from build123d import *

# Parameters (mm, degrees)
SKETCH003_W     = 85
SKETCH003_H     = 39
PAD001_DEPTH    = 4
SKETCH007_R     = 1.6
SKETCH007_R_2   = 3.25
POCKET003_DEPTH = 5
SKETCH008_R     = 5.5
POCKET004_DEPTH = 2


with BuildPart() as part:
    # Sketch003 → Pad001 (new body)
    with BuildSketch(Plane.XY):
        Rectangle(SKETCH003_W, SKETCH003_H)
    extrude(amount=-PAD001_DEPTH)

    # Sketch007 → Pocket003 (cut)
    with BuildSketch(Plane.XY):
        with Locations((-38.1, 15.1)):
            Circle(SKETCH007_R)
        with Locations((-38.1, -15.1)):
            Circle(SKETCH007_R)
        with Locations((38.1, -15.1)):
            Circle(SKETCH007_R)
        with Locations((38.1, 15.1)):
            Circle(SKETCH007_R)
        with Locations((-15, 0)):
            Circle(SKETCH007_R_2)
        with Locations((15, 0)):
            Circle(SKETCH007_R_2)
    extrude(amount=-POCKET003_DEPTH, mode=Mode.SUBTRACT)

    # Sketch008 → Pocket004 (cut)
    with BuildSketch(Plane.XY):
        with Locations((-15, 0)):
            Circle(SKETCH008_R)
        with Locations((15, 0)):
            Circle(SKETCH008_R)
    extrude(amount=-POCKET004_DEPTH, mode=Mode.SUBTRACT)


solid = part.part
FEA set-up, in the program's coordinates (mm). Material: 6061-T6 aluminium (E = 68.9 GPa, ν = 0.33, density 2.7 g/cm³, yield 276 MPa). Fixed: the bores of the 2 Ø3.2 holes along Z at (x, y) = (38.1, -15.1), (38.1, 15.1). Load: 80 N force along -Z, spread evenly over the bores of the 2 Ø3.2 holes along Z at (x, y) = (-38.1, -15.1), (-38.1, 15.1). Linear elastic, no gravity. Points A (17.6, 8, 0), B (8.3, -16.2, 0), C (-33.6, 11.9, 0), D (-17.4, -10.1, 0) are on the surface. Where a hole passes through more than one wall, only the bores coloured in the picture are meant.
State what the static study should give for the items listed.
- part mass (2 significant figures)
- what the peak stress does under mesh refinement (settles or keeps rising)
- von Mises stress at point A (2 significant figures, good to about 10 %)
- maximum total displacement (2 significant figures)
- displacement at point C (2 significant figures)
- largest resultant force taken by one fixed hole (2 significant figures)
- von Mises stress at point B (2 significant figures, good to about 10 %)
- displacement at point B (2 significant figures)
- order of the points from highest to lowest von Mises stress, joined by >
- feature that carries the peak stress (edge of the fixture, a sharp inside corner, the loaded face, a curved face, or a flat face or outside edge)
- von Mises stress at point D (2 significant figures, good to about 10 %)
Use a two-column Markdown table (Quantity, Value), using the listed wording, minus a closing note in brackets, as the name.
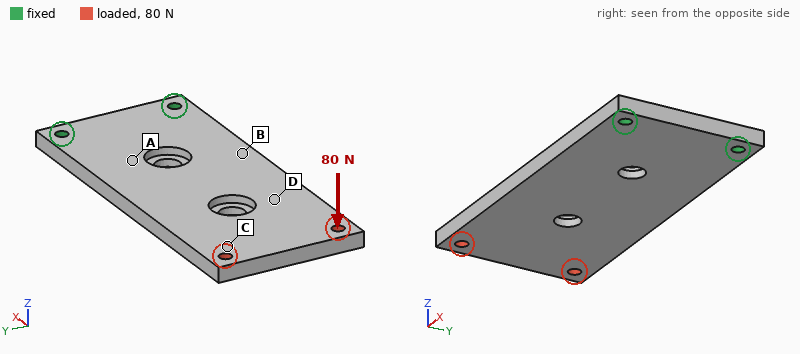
| Quantity | Value |
|---|---|
| part mass | 34 g |
| what the peak stress does under mesh refinement | keeps rising |
| von Mises stress at point A | 57 MPa |
| maximum total displacement | 1.0 mm |
| displacement at point C | 0.88 mm |
| largest resultant force taken by one fixed hole | 44 N |
| von Mises stress at point B | 42 MPa |
| displacement at point B | 0.20 mm |
| order of the points from highest to lowest von Mises stress, joined by > | A > B > D > C |
| feature that carries the peak stress | edge of the fixture |
| von Mises stress at point D | 21 MPa |
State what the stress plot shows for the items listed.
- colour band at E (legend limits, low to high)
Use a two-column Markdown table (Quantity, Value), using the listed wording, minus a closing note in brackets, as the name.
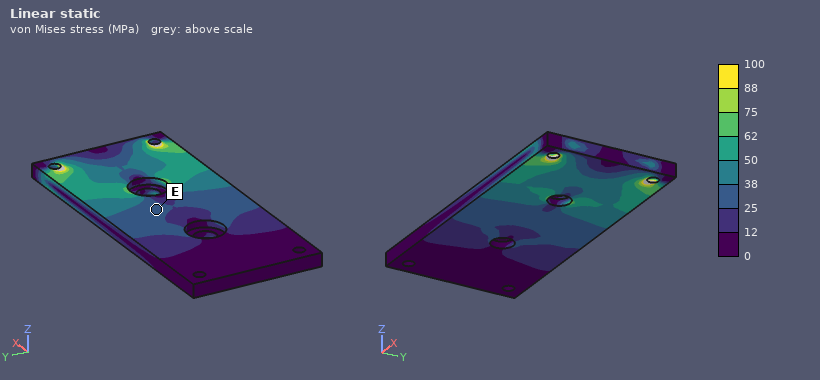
| Quantity | Value |
|---|---|
| colour band at E | 25 to 38 MPa |
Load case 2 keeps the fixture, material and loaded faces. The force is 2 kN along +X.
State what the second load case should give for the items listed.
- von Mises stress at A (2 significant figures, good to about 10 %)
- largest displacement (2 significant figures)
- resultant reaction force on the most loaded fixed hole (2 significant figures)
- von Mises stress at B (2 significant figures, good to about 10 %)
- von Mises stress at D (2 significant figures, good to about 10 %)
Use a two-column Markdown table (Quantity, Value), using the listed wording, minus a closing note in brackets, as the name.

| Quantity | Value |
|---|---|
| von Mises stress at A | 18 MPa |
| largest displacement | 30 µm |
| resultant reaction force on the most loaded fixed hole | 1.0 kN |
| von Mises stress at B | 16 MPa |
| von Mises stress at D | 17 MPa |
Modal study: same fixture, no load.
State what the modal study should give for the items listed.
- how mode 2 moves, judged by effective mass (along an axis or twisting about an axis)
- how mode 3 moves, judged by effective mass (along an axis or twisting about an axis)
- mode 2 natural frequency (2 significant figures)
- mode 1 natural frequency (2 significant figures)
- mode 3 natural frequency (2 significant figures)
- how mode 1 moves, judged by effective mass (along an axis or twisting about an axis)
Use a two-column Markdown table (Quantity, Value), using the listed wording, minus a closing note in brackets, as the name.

| Quantity | Value |
|---|---|
| how mode 2 moves, judged by effective mass | twisting about X |
| how mode 3 moves, judged by effective mass | along Z |
| mode 2 natural frequency | 2100 Hz |
| mode 1 natural frequency | 470 Hz |
| mode 3 natural frequency | 3000 Hz |
| how mode 1 moves, judged by effective mass | along Z |
